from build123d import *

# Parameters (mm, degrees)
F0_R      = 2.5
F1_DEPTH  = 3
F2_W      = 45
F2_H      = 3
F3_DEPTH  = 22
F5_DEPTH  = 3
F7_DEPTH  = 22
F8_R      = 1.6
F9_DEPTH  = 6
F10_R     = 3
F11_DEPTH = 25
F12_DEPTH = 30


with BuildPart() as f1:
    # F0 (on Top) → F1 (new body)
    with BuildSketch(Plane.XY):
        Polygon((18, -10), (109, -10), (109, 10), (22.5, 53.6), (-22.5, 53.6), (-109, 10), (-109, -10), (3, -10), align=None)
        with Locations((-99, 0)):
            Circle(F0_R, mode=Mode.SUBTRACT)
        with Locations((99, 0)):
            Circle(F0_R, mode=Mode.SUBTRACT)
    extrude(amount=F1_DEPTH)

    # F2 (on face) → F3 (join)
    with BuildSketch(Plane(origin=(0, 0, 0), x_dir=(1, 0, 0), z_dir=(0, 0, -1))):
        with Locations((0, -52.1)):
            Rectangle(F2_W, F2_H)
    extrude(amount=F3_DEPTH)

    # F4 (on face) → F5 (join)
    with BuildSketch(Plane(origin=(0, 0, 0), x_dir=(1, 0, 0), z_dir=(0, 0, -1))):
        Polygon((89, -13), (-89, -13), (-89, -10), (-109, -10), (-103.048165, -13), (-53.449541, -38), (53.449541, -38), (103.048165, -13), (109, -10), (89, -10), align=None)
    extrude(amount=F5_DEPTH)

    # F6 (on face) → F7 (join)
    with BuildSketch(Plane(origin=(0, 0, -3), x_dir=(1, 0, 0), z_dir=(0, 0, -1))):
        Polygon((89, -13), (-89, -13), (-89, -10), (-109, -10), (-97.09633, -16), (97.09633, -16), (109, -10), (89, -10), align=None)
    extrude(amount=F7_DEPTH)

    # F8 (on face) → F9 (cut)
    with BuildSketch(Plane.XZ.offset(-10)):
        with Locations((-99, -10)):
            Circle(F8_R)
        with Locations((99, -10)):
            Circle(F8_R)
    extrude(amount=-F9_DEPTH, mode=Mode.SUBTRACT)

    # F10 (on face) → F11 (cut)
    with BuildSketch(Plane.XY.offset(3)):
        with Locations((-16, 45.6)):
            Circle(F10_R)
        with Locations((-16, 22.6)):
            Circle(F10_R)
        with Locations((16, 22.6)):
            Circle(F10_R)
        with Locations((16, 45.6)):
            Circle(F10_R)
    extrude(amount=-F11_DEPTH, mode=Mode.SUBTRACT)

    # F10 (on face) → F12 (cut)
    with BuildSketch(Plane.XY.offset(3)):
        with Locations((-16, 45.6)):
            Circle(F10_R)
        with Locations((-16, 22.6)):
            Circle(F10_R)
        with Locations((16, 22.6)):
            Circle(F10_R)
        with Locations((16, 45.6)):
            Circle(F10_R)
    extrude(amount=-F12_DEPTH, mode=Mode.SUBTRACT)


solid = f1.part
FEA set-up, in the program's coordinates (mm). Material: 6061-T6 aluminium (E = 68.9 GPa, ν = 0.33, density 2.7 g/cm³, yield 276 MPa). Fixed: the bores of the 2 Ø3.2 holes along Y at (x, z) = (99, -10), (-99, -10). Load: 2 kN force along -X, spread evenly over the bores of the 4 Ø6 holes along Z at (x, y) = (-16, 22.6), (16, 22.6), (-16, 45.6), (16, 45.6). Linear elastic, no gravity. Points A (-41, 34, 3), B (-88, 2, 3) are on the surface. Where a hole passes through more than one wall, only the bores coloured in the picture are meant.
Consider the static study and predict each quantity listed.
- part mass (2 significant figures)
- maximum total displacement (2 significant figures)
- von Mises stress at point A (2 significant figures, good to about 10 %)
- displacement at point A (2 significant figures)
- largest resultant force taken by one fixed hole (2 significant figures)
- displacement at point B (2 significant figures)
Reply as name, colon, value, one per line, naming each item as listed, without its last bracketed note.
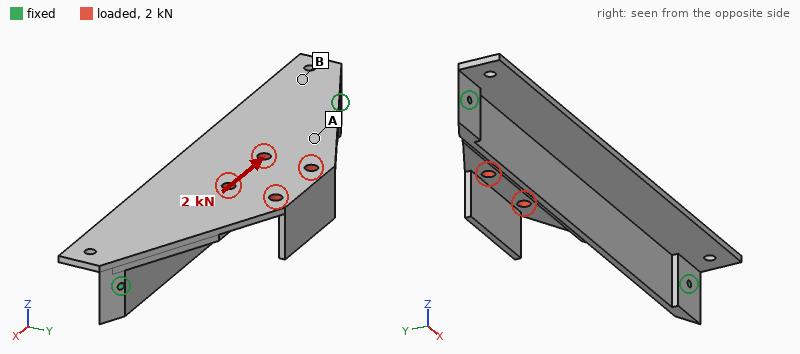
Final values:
part mass: 160 g
maximum total displacement: 18 µm
von Mises stress at point A: 3.8 MPa
displacement at point A: 11 µm
largest resultant force taken by one fixed hole: 1.0 kN
displacement at point B: 8.4 µm
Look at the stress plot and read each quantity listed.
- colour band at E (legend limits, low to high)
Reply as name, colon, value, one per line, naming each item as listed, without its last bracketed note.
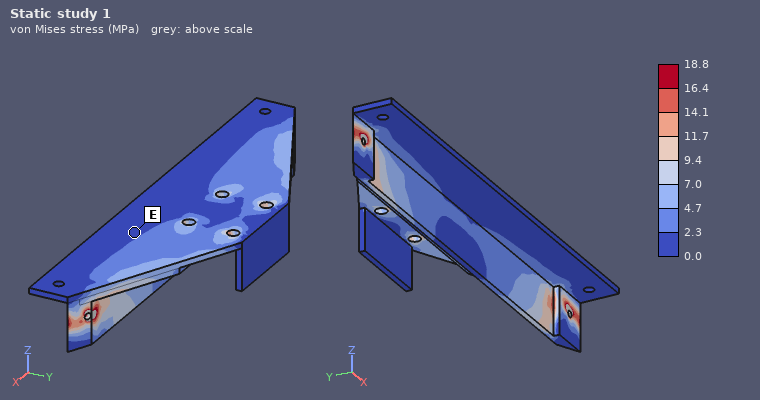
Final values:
colour band at E: 0.0 to 2.3 MPa
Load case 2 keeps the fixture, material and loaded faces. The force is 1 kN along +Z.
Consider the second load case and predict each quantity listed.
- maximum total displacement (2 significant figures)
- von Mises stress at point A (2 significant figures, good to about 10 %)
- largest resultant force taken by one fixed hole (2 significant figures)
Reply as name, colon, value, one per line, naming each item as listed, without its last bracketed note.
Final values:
maximum total displacement: 0.84 mm
von Mises stress at point A: 32 MPa
largest resultant force taken by one fixed hole: 1.2 kN
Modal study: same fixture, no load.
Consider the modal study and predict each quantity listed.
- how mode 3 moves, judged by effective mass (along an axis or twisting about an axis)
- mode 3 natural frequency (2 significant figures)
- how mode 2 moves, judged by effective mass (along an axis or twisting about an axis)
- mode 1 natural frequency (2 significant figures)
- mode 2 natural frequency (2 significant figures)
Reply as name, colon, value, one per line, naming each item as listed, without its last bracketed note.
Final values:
how mode 3 moves, judged by effective mass: along Y
mode 3 natural frequency: 2000 Hz
how mode 2 moves, judged by effective mass: along Z
mode 1 natural frequency: 770 Hz
mode 2 natural frequency: 1600 Hz
